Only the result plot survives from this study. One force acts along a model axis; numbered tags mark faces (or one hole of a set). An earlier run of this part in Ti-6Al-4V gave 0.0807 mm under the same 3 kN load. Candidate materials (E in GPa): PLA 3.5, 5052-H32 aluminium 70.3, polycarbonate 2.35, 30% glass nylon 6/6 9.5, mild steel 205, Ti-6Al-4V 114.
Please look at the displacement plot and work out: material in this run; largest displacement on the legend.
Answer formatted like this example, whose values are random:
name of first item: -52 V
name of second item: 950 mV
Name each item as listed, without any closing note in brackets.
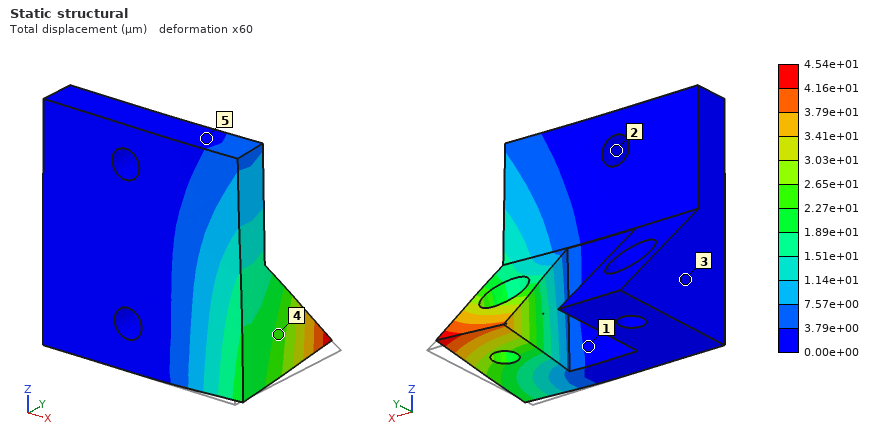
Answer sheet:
material in this run: mild steel
largest displacement on the legend: 4.54e+01 µm
